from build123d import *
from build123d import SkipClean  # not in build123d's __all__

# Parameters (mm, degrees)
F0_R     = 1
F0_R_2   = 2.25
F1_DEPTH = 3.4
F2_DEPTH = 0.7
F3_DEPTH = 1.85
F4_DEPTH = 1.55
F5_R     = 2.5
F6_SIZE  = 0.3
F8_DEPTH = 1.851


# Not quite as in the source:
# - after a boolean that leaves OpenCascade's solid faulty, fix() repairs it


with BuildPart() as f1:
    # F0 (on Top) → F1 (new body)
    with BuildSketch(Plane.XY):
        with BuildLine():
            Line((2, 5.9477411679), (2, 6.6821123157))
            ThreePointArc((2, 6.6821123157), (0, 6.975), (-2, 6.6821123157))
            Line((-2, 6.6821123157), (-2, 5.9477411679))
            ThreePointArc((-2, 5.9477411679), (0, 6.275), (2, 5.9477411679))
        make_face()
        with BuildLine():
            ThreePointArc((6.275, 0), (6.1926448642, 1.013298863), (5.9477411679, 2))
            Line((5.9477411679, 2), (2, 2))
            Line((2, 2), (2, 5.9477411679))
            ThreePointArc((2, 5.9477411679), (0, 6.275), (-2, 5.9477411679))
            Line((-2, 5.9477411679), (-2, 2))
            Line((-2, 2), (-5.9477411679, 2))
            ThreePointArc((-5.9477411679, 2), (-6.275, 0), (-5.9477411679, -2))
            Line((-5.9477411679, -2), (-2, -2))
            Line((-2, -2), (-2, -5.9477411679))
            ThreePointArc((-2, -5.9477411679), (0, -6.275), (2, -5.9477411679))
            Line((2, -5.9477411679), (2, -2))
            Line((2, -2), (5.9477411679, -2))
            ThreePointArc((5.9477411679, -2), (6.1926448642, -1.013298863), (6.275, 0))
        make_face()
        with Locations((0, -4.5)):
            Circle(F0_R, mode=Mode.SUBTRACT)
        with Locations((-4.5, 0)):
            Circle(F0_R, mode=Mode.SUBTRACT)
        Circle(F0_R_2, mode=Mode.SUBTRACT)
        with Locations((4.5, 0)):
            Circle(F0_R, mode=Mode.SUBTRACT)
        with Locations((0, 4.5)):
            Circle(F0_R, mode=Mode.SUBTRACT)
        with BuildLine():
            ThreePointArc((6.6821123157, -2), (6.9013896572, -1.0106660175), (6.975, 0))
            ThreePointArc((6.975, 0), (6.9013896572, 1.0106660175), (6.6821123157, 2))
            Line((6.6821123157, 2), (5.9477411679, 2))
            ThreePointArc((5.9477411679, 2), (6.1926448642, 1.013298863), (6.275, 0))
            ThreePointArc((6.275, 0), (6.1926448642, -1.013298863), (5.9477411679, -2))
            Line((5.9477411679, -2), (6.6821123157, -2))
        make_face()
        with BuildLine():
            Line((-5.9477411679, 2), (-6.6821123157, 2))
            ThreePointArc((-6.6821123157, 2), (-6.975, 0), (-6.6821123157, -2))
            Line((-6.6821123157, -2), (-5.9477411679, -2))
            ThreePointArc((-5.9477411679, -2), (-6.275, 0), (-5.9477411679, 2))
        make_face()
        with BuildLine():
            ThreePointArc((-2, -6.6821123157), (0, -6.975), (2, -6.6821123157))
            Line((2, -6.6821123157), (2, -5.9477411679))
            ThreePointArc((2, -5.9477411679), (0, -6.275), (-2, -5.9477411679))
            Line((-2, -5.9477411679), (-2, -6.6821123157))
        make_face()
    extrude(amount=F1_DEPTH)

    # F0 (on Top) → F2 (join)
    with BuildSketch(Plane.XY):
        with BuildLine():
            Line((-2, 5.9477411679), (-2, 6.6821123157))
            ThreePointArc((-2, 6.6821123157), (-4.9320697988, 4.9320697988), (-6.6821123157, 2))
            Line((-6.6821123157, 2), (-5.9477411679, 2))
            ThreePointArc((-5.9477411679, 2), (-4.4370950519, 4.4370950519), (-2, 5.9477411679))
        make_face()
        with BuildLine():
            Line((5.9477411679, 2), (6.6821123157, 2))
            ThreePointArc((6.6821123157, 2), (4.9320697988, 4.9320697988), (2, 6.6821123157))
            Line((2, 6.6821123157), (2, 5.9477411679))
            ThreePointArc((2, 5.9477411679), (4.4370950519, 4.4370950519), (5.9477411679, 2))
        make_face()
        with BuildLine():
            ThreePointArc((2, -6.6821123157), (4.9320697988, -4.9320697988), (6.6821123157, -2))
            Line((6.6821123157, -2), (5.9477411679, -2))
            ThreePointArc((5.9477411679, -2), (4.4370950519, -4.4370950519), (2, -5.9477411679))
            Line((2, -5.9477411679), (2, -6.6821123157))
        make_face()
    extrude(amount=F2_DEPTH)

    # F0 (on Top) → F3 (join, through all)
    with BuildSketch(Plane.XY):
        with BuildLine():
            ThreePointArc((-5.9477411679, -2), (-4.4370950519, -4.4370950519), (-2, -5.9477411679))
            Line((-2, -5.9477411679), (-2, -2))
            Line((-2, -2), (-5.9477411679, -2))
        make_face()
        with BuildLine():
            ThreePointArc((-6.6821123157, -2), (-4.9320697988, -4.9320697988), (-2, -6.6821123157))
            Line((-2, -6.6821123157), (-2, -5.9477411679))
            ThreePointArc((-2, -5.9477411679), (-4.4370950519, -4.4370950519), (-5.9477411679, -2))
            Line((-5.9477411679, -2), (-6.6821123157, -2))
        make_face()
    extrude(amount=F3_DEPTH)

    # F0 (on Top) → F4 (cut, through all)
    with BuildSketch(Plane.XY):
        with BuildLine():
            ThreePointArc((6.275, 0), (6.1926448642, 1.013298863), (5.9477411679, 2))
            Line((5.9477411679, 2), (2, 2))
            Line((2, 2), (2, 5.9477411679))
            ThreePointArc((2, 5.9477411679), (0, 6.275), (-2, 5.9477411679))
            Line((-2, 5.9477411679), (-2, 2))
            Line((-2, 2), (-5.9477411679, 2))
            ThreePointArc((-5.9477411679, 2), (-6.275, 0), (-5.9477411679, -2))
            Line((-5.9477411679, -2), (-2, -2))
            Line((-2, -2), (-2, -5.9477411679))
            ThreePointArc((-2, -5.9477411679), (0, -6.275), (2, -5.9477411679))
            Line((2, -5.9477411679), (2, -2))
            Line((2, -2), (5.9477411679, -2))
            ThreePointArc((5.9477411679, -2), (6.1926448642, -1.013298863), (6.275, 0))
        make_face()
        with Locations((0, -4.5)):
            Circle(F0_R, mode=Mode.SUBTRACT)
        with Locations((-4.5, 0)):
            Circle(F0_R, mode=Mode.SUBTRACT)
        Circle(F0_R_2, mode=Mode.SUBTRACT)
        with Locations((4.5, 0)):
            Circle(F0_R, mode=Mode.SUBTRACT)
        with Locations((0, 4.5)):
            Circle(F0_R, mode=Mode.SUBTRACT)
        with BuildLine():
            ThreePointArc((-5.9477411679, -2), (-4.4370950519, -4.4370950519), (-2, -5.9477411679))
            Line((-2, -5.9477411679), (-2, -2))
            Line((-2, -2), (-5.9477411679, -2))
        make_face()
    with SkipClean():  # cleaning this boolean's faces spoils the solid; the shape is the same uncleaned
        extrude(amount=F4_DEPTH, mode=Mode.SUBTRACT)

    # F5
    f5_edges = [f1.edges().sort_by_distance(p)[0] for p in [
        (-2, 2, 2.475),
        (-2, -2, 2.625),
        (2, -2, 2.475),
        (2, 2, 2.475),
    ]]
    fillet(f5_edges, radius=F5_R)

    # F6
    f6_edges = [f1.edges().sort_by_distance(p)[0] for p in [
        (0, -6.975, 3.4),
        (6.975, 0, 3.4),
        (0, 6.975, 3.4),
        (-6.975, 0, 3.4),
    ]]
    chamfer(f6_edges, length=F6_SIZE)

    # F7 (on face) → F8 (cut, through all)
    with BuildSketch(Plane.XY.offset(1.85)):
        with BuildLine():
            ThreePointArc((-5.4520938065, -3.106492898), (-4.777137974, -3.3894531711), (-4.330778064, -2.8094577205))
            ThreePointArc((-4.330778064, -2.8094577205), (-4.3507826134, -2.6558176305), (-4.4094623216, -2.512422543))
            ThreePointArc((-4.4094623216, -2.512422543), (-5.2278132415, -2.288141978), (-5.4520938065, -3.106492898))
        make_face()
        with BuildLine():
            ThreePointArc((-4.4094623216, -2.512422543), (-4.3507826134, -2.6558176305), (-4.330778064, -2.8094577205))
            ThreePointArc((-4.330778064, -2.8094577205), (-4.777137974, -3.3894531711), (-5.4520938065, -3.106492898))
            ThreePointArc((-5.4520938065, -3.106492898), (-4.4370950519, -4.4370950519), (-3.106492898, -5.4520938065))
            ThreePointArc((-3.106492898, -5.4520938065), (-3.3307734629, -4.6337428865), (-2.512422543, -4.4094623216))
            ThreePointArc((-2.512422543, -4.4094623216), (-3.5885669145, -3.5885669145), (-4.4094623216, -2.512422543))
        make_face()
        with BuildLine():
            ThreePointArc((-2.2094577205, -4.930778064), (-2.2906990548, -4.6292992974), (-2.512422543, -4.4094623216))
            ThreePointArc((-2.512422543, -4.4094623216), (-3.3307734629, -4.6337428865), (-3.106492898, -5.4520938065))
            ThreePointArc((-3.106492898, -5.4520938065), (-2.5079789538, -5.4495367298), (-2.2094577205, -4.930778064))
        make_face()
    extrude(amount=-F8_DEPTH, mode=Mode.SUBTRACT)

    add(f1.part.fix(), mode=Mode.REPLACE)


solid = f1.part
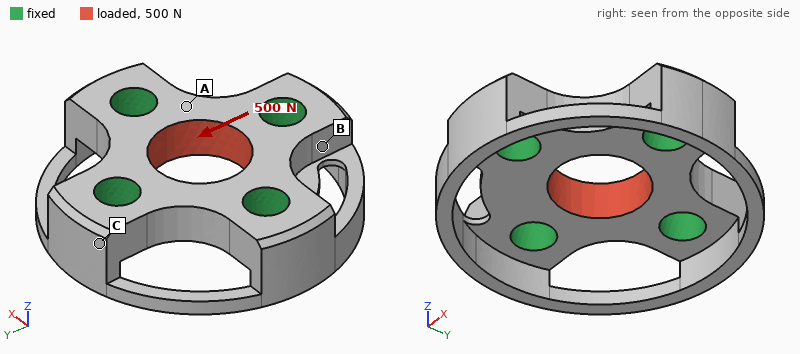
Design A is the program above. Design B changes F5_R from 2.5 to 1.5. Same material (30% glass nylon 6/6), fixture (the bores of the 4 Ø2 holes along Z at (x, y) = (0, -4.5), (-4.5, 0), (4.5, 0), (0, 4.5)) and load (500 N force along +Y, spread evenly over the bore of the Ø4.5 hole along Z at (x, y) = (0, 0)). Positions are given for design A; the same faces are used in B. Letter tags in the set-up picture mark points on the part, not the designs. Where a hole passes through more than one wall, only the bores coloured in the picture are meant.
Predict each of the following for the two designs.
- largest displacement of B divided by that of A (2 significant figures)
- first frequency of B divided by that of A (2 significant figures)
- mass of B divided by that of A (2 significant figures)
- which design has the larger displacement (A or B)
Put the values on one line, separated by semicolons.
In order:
1.1; 1.00; 0.96; B
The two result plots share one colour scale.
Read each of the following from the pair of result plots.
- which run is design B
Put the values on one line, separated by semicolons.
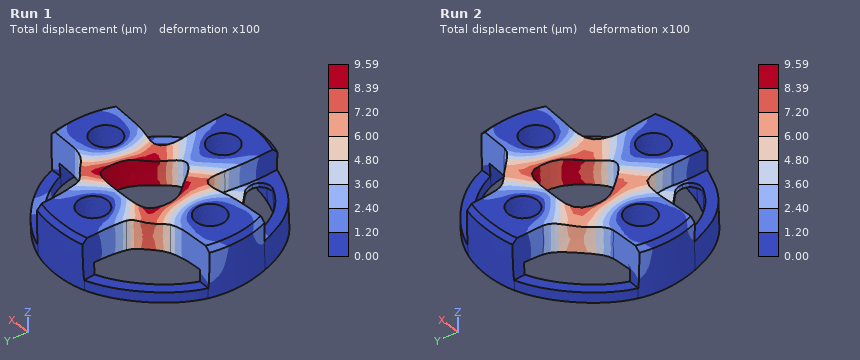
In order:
Run 1
